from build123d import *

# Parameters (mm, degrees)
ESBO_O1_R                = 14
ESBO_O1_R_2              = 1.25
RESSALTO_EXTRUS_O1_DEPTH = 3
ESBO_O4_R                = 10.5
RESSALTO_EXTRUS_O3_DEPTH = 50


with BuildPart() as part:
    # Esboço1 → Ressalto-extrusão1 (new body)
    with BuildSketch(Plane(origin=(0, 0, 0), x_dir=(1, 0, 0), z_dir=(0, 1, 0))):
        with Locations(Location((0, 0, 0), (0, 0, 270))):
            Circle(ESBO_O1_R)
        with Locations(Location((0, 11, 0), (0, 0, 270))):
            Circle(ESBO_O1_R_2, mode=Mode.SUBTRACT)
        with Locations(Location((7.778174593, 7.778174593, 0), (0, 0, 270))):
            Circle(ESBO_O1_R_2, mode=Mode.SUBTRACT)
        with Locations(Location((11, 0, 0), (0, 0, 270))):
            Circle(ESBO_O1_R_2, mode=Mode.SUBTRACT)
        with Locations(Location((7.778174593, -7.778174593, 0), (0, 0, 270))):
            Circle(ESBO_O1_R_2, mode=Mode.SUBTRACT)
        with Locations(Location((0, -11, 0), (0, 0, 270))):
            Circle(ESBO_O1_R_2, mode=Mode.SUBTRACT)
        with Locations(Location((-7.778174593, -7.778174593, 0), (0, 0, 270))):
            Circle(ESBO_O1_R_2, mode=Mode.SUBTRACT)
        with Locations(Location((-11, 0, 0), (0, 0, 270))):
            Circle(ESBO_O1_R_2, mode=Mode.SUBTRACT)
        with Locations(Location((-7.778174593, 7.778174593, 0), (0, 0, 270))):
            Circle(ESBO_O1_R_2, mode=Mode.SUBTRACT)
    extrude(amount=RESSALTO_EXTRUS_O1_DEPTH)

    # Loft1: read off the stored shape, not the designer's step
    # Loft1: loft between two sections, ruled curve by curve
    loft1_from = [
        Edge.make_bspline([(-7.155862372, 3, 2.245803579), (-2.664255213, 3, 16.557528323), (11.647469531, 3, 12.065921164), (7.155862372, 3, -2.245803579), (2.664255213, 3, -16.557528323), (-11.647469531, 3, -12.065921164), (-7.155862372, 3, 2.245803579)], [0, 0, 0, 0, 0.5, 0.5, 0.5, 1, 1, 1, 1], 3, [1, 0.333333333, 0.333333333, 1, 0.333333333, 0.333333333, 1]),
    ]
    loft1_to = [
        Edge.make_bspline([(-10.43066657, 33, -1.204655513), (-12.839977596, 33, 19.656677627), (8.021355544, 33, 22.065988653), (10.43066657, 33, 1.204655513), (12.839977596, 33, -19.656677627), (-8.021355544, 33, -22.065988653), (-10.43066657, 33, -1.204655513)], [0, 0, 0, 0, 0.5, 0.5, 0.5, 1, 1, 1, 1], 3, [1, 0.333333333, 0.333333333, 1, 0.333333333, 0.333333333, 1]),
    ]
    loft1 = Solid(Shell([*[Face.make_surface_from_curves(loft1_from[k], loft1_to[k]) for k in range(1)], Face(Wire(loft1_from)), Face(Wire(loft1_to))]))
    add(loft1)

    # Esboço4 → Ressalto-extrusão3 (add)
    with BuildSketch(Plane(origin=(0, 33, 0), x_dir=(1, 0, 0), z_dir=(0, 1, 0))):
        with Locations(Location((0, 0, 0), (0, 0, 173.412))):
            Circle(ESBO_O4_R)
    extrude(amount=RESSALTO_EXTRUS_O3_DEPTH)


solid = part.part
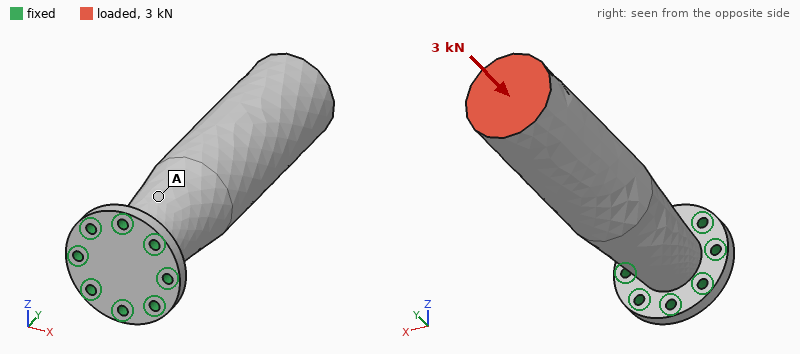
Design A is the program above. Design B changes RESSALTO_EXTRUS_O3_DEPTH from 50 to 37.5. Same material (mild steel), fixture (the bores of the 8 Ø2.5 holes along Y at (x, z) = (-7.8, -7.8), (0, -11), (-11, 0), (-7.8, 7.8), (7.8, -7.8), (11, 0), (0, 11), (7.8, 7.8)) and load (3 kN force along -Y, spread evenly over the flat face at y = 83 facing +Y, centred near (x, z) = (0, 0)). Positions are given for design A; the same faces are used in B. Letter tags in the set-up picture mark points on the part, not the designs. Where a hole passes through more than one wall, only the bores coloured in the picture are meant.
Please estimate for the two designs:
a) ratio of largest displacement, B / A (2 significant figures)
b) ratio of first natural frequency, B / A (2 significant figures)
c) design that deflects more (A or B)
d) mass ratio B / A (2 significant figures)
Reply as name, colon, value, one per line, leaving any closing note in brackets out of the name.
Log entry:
ratio of largest displacement, B / A: 0.91
ratio of first natural frequency, B / A: 1.3
design that deflects more: A
mass ratio B / A: 0.84
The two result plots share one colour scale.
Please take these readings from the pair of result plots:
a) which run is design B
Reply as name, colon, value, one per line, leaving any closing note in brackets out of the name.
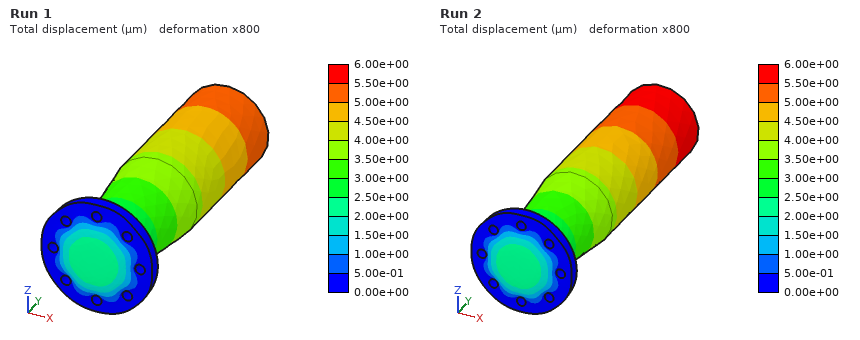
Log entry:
which run is design B: Run 1
